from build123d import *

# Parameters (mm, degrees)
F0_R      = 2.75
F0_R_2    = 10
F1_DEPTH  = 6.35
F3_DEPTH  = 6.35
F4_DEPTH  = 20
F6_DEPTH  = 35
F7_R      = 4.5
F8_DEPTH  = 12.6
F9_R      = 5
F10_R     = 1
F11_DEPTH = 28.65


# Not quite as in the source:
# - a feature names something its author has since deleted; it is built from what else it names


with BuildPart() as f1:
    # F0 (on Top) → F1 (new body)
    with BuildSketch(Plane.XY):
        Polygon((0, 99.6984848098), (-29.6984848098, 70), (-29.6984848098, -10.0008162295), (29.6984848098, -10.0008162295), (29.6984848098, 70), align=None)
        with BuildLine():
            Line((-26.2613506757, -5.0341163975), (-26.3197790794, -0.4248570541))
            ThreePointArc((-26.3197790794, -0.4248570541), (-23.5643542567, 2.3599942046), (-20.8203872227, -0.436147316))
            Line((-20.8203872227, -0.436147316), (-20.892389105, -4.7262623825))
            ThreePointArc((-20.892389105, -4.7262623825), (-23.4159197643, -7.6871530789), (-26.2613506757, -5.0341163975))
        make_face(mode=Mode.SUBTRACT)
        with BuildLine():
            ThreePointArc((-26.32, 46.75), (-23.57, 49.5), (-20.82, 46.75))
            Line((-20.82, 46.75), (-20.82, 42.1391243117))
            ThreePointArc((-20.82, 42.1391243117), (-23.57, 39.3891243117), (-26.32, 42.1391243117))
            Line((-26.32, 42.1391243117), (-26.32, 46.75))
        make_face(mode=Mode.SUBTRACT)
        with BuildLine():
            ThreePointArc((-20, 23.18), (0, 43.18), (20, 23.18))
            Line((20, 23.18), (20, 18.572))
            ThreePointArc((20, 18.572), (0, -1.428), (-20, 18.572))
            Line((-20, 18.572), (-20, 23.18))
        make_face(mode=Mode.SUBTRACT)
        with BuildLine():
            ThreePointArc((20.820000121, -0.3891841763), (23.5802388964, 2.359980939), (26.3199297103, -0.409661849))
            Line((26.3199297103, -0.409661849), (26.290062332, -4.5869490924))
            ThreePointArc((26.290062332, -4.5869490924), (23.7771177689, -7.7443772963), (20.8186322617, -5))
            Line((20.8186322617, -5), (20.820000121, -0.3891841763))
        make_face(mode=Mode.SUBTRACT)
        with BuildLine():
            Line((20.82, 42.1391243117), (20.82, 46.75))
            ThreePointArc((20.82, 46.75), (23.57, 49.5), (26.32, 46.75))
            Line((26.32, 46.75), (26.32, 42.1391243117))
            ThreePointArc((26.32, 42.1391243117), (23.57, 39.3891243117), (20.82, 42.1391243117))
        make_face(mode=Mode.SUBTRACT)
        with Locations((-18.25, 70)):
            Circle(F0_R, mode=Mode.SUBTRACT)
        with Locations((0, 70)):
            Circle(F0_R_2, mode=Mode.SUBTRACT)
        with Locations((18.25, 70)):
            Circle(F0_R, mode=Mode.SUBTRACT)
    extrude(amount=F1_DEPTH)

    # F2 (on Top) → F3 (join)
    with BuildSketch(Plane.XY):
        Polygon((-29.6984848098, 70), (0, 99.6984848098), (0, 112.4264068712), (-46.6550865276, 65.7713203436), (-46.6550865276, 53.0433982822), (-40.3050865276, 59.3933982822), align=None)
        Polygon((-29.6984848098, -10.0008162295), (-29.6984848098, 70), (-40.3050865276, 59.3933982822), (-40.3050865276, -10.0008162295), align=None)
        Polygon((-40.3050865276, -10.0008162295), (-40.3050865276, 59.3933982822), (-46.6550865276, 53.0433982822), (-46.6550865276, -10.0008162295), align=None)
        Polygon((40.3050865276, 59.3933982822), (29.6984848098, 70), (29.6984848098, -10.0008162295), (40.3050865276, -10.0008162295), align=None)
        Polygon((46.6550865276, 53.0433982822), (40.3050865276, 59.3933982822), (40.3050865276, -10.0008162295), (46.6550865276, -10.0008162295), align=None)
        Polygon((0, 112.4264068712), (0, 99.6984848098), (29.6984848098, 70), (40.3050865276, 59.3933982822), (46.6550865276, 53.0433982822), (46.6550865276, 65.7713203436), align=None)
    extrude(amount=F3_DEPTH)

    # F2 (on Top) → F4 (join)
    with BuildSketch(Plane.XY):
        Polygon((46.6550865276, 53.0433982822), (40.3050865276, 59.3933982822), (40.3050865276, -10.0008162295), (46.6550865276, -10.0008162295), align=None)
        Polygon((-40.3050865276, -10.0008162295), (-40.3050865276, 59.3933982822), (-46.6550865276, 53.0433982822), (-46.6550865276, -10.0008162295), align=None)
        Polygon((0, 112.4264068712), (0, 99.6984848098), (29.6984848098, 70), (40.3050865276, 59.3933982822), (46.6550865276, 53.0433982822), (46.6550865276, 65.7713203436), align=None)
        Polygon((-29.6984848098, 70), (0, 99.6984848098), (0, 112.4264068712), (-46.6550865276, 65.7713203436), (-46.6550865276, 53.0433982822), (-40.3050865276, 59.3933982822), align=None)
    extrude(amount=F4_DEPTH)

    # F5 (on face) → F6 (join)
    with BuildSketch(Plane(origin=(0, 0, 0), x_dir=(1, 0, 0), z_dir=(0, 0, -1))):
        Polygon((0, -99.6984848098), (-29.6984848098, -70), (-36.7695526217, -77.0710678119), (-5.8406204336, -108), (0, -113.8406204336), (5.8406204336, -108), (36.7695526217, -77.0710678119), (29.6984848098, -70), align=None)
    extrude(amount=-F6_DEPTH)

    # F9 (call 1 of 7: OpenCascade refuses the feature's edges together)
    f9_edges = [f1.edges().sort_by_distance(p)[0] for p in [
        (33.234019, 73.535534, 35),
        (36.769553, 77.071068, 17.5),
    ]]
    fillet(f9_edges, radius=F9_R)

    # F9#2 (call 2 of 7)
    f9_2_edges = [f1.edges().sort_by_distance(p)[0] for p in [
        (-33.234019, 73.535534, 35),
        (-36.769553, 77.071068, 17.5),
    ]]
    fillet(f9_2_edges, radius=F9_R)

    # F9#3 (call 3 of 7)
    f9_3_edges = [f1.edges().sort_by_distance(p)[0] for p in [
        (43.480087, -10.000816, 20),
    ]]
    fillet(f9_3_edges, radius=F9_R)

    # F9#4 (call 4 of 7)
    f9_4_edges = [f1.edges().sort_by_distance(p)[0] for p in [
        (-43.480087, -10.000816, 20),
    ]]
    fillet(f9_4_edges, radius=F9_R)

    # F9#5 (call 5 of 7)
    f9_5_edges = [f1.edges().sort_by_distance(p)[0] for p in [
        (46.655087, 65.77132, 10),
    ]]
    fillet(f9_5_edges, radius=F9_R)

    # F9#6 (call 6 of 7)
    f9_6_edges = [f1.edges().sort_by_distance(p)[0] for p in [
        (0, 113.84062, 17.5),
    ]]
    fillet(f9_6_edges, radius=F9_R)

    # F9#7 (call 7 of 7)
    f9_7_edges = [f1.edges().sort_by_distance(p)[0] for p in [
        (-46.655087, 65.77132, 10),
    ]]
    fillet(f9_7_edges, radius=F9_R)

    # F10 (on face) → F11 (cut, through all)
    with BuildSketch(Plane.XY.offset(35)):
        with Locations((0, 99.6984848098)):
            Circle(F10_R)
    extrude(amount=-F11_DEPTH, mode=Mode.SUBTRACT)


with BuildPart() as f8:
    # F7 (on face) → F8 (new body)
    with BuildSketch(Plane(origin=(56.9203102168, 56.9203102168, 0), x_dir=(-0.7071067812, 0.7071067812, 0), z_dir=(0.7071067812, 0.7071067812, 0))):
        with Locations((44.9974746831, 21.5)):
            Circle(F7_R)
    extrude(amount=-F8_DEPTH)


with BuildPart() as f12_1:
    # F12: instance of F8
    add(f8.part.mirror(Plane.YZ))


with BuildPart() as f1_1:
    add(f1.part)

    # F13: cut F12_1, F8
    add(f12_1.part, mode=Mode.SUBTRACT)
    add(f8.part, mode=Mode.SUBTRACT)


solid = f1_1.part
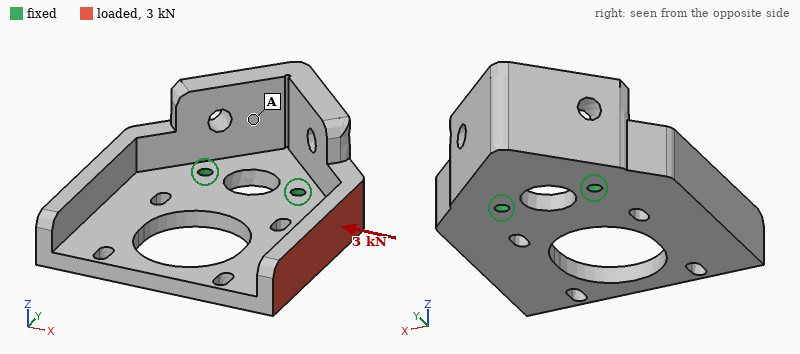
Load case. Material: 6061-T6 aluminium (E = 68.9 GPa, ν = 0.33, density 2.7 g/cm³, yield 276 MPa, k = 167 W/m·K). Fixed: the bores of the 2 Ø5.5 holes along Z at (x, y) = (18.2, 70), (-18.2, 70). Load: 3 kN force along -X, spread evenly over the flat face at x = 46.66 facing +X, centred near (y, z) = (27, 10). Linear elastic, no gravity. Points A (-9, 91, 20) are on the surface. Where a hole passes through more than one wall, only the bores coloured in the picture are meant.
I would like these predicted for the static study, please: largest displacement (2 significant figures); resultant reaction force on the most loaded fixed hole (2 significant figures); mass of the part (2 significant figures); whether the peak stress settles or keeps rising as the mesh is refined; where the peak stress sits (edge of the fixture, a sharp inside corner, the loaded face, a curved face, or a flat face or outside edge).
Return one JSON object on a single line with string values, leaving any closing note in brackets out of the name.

{"largest displacement": "0.23 mm", "resultant reaction force on the most loaded fixed hole": "3.4 kN", "mass of the part": "240 g", "whether the peak stress settles or keeps rising as the mesh is refined": "keeps rising", "where the peak stress sits": "edge of the fixture"}
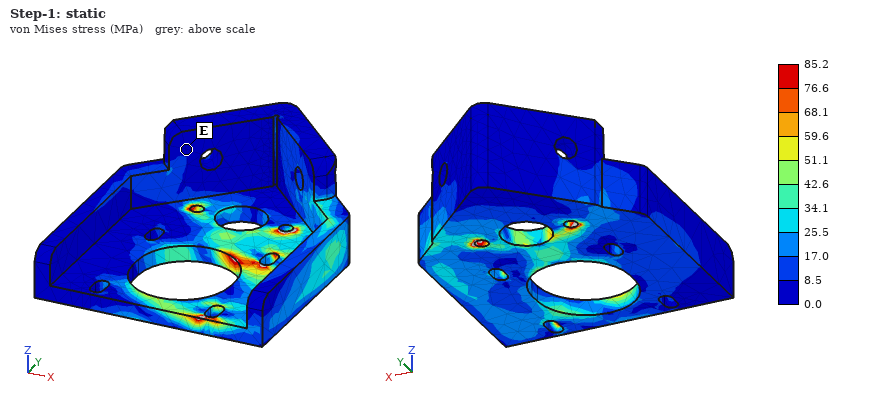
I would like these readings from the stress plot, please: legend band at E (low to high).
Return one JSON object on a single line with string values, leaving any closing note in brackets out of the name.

{"legend band at E": "0.0 to 8.5 MPa"}
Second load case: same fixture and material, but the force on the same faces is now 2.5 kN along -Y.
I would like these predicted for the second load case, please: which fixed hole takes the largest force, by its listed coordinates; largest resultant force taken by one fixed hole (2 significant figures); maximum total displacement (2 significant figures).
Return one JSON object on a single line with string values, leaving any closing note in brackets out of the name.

{"which fixed hole takes the largest force, by its listed coordinates": "(18.2, 70)", "largest resultant force taken by one fixed hole": "4.1 kN", "maximum total displacement": "0.15 mm"}
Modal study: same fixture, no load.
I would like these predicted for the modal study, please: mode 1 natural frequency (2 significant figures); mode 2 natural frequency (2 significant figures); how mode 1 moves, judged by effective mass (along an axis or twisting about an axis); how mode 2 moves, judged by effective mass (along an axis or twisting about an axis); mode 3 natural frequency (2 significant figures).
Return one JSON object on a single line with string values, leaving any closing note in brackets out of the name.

{"mode 1 natural frequency": "970 Hz", "mode 2 natural frequency": "1800 Hz", "how mode 1 moves, judged by effective mass": "along Z", "how mode 2 moves, judged by effective mass": "twisting about Y", "mode 3 natural frequency": "2700 Hz"}
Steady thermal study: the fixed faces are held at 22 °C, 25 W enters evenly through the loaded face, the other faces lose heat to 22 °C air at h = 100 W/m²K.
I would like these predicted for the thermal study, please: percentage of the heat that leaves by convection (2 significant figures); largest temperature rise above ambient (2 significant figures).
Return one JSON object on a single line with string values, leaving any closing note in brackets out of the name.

{"percentage of the heat that leaves by convection": "44 %", "largest temperature rise above ambient": "17 K"}
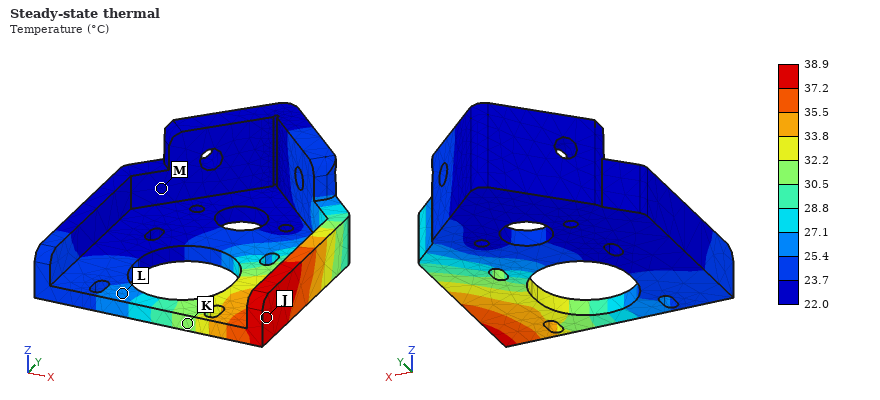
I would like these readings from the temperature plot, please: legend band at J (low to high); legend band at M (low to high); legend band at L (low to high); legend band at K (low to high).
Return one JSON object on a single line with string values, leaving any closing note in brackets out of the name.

{"legend band at J": "37.2 to 38.9 °C", "legend band at M": "22.0 to 23.7 °C", "legend band at L": "25.4 to 27.1 °C", "legend band at K": "30.5 to 32.2 °C"}
